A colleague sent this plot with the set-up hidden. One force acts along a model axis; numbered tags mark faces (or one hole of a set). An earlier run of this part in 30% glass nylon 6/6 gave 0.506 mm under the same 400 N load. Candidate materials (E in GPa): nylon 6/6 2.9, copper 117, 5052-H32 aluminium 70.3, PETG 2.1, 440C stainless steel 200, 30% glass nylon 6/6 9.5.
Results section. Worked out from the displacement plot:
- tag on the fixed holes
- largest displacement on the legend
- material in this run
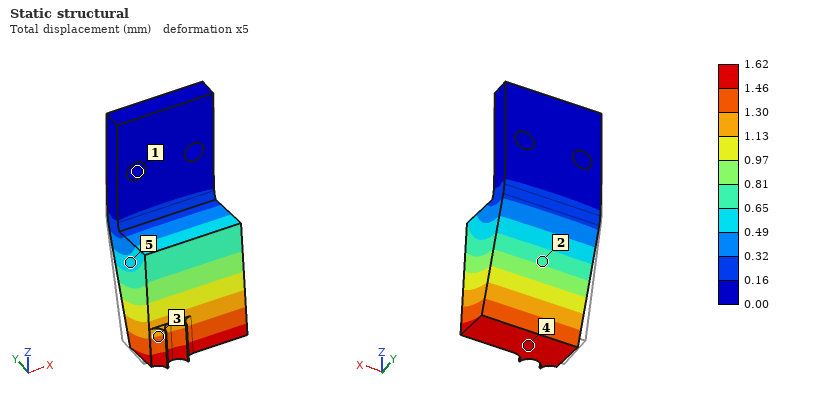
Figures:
1
1.62 mm
nylon 6/6
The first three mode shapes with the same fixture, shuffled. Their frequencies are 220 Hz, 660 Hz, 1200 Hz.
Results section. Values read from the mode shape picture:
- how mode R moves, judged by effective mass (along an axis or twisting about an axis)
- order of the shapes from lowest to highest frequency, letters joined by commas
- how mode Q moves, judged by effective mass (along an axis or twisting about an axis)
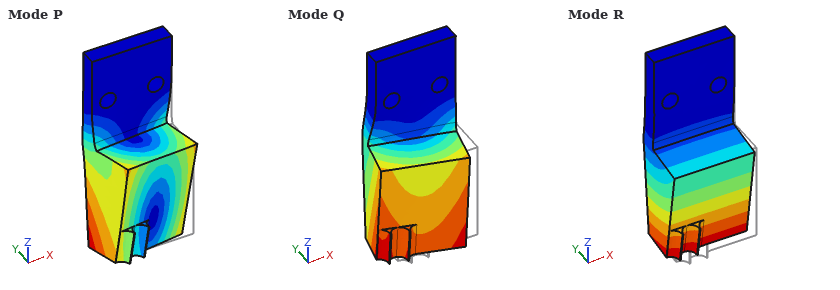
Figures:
along Y
R, Q, P
along X
